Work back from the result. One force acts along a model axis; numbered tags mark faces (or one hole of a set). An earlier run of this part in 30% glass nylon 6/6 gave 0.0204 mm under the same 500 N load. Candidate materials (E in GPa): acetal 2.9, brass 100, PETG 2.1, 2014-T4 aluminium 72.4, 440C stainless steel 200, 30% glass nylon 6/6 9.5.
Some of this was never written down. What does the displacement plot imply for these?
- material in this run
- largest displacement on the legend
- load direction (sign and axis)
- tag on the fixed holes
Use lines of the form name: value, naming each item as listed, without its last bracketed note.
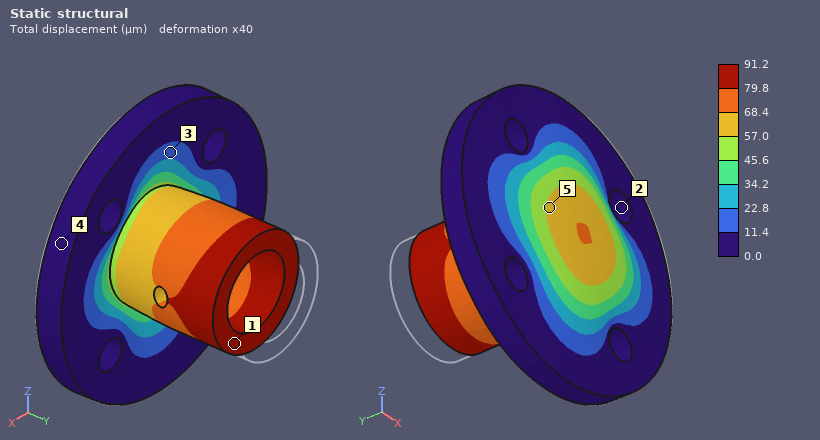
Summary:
material in this run: PETG
largest displacement on the legend: 91.2 µm
load direction: -Y
tag on the fixed holes: 2
